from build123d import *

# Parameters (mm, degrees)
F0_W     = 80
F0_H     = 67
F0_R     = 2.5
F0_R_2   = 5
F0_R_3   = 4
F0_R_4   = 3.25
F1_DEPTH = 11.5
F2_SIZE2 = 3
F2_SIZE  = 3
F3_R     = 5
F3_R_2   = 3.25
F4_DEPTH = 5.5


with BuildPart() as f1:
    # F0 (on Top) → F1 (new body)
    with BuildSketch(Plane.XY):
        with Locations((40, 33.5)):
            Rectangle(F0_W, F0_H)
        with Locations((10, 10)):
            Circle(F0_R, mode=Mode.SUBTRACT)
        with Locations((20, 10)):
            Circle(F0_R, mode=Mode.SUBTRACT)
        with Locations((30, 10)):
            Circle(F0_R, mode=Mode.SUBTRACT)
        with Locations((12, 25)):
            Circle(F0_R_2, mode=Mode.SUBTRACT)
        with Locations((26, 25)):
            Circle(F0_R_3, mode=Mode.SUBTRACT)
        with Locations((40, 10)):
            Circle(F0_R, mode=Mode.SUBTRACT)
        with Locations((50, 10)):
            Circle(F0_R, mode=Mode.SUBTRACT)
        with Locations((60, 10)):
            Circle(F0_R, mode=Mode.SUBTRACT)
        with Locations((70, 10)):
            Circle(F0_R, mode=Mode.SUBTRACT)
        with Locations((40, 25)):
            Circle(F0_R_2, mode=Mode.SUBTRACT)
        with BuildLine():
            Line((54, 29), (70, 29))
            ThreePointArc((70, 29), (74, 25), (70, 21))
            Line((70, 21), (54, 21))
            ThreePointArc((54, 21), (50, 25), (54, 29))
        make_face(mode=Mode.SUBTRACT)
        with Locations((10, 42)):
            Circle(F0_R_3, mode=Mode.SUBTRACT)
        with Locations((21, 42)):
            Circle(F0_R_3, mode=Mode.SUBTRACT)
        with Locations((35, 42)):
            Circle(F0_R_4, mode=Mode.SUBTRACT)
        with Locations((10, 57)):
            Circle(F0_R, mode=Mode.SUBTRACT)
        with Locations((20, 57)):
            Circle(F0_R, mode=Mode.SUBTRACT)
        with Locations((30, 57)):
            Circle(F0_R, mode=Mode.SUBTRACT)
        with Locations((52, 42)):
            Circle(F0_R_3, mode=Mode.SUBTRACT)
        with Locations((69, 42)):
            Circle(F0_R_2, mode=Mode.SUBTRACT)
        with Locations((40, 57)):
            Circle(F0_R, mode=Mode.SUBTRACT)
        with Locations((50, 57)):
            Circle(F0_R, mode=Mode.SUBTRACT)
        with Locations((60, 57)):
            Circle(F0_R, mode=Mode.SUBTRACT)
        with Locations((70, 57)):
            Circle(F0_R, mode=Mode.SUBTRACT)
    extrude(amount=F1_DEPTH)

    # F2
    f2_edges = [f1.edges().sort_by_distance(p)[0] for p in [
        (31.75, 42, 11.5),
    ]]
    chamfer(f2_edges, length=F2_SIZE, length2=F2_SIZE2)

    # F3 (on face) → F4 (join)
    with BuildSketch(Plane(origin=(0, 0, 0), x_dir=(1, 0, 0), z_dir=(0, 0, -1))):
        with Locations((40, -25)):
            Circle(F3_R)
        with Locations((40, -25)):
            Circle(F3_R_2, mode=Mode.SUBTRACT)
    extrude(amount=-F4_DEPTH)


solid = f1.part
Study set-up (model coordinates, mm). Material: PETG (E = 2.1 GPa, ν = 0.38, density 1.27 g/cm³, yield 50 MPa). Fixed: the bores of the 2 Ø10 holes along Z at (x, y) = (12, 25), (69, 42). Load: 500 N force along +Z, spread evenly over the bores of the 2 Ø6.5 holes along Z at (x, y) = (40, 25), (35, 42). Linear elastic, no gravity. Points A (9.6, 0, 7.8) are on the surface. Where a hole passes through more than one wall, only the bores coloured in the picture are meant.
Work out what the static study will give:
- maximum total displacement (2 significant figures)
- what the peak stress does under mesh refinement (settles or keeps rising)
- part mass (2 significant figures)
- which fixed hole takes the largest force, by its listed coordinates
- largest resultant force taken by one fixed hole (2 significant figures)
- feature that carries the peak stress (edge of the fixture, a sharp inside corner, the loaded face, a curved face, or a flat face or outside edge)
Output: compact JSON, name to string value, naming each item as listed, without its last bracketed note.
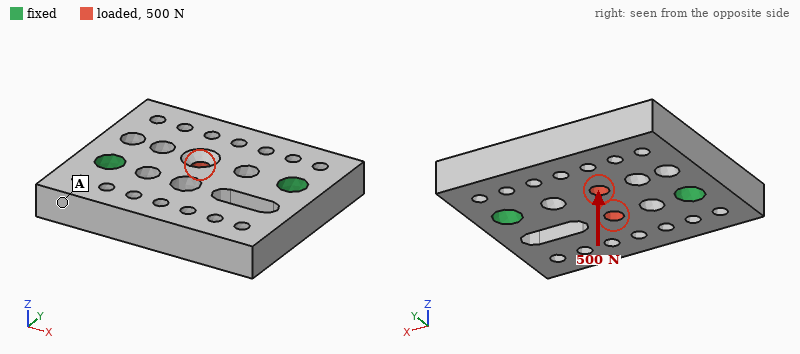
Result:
{"maximum total displacement": "99 µm", "what the peak stress does under mesh refinement": "keeps rising", "part mass": "65 g", "which fixed hole takes the largest force, by its listed coordinates": "(12, 25)", "largest resultant force taken by one fixed hole": "290 N", "feature that carries the peak stress": "a sharp inside corner"}
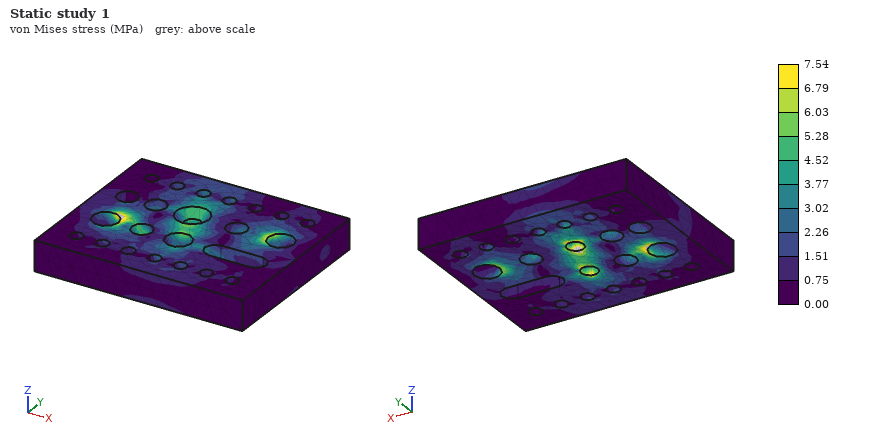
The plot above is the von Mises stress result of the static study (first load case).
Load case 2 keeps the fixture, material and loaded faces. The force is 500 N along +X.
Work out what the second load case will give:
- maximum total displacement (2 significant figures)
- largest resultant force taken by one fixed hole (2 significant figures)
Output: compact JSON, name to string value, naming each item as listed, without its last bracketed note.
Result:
{"maximum total displacement": "21 µm", "largest resultant force taken by one fixed hole": "260 N"}
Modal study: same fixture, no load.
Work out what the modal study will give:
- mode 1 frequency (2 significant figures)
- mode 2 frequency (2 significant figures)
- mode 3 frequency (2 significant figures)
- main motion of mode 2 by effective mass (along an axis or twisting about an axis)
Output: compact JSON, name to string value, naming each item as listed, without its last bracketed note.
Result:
{"mode 1 frequency": "1300 Hz", "mode 2 frequency": "1500 Hz", "mode 3 frequency": "2900 Hz", "main motion of mode 2 by effective mass": "along Z"}
